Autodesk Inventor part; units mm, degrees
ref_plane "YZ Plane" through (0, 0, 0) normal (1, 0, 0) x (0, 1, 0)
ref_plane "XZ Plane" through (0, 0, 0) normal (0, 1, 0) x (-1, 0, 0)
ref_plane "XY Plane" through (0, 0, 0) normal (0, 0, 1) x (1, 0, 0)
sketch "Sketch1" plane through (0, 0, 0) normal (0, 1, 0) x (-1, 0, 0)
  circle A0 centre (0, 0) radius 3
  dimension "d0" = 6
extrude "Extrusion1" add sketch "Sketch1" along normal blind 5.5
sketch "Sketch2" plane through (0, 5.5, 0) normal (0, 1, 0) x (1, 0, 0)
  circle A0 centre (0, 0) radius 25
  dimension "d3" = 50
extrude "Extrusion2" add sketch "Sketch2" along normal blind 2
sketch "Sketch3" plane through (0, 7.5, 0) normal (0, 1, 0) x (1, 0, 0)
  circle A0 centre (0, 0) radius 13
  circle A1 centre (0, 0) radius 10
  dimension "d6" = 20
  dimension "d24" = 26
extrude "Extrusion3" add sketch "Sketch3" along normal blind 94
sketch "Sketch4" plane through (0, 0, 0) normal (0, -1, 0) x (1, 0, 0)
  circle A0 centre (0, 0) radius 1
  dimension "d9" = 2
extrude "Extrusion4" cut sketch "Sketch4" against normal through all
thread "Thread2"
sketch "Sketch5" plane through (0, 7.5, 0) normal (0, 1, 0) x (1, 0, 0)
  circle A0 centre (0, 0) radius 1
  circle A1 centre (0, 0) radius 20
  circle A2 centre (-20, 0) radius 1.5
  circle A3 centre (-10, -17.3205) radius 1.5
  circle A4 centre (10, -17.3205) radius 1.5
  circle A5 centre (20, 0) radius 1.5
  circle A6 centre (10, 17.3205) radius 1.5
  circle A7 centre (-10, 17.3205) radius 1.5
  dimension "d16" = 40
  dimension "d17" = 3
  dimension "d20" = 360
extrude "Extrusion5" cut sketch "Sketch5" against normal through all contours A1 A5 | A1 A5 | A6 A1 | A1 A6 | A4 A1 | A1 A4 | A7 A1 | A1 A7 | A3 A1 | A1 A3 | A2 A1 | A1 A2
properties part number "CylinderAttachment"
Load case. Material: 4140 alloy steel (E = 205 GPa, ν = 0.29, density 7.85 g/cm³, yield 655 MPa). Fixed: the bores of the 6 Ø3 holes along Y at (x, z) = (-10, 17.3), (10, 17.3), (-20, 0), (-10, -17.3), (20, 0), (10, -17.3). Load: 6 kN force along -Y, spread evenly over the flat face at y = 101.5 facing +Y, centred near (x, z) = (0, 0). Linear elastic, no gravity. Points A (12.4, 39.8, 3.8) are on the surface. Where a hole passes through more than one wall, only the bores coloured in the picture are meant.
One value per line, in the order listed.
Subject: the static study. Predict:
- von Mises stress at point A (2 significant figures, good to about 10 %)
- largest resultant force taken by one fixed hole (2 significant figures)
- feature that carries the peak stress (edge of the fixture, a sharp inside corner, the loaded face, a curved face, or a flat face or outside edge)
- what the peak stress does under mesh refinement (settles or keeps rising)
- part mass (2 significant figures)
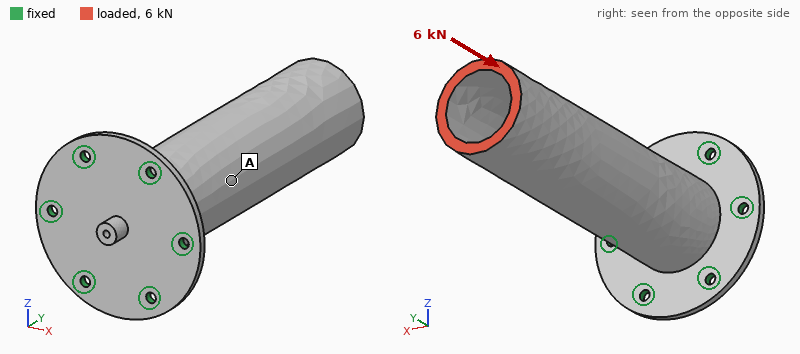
28 MPa
1.1 kN
edge of the fixture
keeps rising
190 g
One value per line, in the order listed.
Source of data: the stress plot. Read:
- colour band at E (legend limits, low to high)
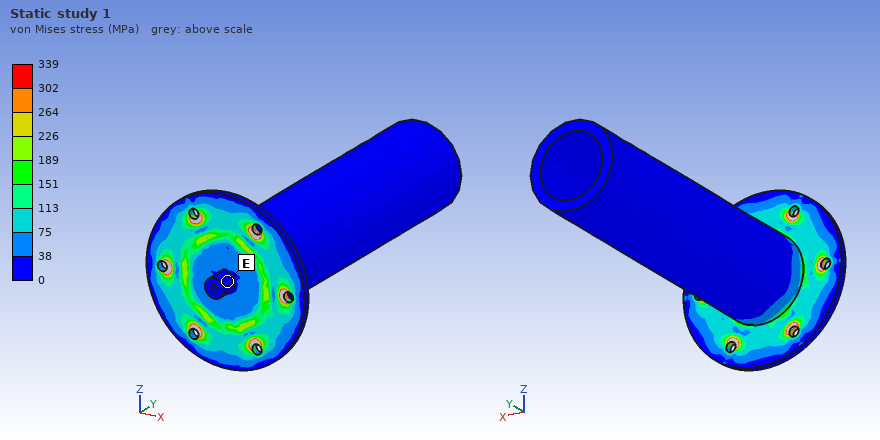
0 to 38 MPa
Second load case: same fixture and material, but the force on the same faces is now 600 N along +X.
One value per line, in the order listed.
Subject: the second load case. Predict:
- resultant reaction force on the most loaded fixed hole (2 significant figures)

1.2 kN
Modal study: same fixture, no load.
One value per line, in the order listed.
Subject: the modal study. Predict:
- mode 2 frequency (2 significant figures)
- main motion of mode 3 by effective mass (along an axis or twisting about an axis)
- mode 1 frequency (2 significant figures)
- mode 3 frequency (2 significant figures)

1100 Hz
along Y
1100 Hz
5200 Hz
